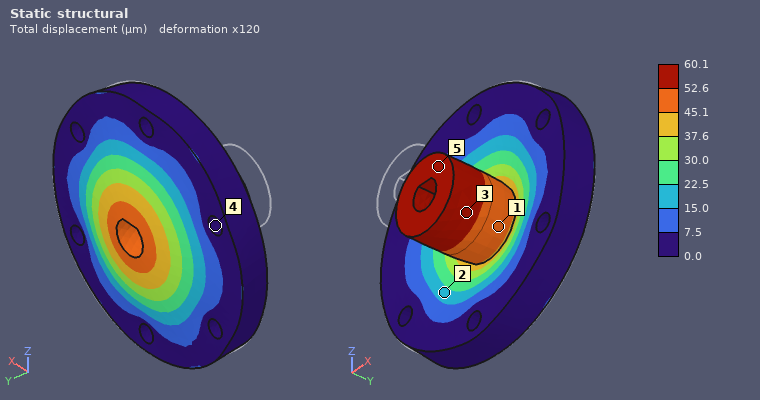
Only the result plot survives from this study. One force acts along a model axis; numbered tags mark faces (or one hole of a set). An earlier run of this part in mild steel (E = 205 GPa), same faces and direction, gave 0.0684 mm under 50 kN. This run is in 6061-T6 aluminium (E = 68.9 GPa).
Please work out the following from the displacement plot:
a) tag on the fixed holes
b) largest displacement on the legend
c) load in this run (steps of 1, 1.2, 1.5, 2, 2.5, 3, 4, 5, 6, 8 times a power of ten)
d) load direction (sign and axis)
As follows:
4
60.1 µm
15 kN
+Y
